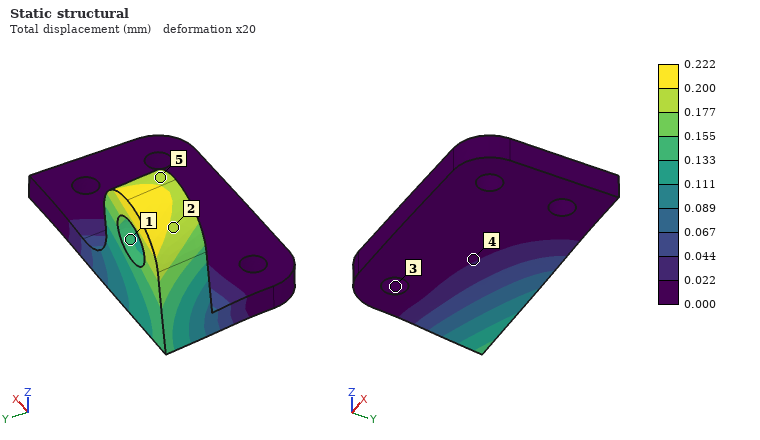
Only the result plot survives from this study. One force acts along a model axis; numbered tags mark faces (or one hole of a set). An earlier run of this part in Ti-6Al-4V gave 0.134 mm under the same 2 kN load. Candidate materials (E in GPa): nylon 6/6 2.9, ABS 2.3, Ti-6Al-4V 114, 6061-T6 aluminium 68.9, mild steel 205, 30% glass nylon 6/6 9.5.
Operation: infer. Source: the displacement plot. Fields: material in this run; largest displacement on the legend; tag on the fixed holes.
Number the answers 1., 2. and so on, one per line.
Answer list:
1. 6061-T6 aluminium
2. 0.222 mm
3. 3
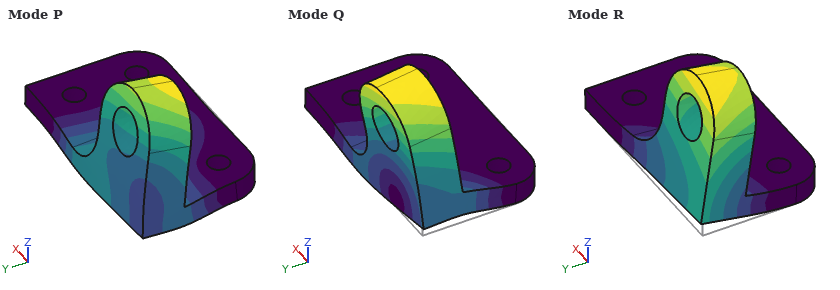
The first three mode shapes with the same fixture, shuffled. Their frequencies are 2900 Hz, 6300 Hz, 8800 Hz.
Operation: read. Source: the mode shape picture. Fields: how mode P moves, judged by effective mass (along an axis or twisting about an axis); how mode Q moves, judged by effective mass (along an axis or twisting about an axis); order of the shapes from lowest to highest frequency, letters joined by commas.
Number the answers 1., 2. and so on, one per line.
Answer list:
1. along Z
2. along X
3. R, Q, P
